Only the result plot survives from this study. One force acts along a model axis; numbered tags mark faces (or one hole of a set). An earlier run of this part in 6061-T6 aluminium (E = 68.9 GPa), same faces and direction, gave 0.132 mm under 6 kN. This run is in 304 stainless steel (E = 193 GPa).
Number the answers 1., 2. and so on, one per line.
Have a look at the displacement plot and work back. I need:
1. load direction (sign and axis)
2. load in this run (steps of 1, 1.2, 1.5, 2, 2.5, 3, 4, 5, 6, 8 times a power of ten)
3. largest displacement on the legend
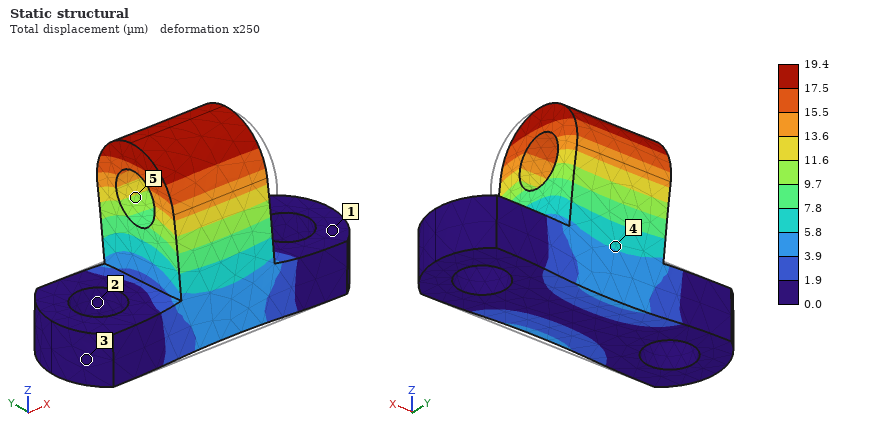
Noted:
1. +Y
2. 2.5 kN
3. 19.4 µm
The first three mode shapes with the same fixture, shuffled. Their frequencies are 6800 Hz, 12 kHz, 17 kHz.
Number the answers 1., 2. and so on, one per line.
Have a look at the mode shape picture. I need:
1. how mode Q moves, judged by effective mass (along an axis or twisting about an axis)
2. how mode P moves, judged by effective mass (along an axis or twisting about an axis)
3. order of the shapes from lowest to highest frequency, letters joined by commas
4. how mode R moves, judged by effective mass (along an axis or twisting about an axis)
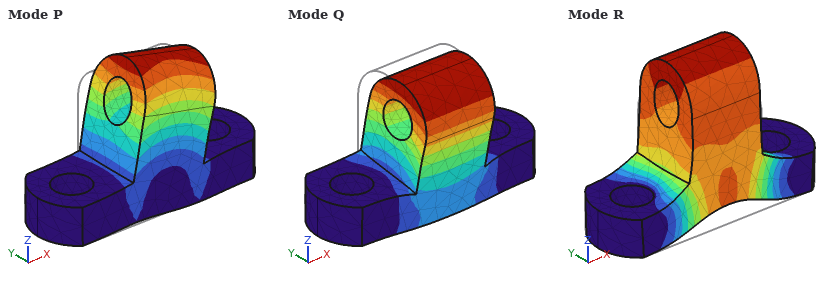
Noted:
1. along Y
2. along X
3. Q, P, R
4. along Z
